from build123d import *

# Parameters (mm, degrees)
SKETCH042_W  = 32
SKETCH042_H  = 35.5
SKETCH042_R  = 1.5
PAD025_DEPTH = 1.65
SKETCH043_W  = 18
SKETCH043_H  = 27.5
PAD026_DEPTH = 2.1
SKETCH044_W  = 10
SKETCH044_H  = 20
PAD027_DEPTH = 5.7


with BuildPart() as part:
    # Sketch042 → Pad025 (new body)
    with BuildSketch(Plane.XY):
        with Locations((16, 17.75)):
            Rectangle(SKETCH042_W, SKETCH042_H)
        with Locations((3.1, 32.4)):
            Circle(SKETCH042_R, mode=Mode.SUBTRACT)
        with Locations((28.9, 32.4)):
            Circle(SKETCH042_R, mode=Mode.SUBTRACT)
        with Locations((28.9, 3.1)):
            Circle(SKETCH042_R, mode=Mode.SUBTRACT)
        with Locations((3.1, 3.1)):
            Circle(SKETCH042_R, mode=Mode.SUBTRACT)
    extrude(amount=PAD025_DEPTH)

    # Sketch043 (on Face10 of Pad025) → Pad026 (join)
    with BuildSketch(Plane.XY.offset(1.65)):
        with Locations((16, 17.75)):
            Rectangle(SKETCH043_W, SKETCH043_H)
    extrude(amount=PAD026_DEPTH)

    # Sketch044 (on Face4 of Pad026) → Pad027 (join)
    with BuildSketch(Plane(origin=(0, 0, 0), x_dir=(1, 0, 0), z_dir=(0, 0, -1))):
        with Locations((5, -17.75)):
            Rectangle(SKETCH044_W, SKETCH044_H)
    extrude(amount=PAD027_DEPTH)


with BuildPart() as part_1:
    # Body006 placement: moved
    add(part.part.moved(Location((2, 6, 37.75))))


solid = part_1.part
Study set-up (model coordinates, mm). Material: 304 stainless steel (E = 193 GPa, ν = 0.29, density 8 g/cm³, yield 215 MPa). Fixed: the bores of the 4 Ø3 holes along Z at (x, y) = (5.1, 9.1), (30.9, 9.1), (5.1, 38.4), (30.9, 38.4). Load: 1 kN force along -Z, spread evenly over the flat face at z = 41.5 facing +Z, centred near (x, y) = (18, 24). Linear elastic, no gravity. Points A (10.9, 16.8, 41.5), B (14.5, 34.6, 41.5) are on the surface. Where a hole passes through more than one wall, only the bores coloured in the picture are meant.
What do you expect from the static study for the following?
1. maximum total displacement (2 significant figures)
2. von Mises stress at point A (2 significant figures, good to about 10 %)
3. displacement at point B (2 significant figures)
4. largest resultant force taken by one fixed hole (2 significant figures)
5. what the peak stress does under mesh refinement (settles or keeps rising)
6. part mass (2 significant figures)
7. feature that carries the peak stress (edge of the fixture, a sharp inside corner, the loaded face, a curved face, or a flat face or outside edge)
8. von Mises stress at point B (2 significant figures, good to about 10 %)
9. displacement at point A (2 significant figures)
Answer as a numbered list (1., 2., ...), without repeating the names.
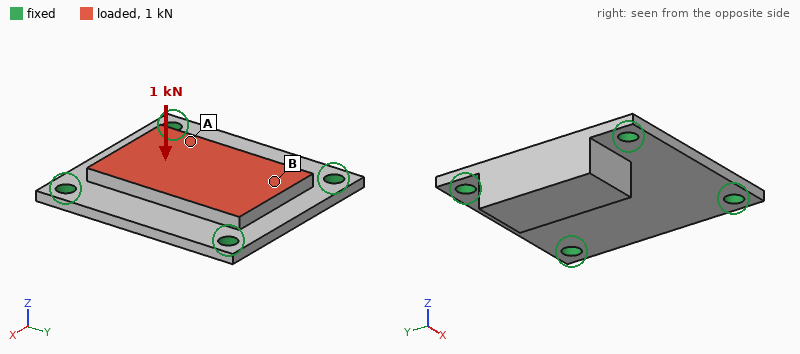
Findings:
1. 13 µm
2. 17 MPa
3. 8.7 µm
4. 340 N
5. keeps rising
6. 32 g
7. edge of the fixture
8. 33 MPa
9. 7.7 µm
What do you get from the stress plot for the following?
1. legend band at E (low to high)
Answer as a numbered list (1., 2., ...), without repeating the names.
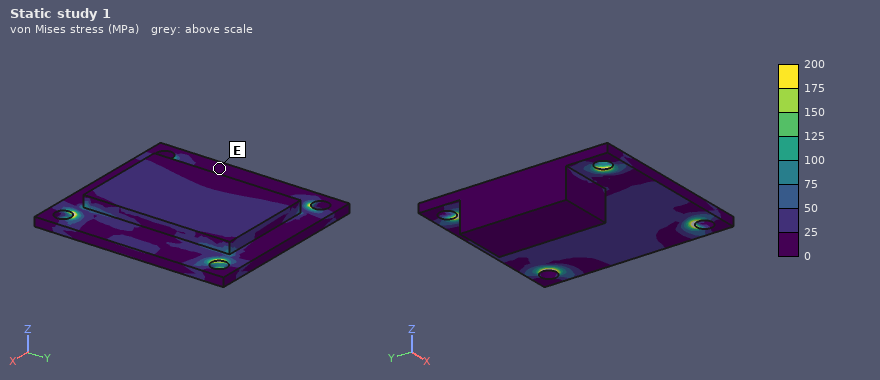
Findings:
1. 0 to 25 MPa
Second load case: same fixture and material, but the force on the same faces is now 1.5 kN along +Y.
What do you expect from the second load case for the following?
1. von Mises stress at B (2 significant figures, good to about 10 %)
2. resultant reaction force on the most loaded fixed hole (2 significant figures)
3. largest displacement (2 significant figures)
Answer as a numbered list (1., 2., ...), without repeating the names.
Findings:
1. 15 MPa
2. 430 N
3. 3.9 µm
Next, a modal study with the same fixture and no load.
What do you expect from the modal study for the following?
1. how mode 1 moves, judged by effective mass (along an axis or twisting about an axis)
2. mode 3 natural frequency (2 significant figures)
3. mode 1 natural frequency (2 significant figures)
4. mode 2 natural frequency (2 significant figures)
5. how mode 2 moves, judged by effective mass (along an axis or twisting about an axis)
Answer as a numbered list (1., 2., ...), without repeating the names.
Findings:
1. along Z
2. 19 kHz
3. 11 kHz
4. 15 kHz
5. along Z
